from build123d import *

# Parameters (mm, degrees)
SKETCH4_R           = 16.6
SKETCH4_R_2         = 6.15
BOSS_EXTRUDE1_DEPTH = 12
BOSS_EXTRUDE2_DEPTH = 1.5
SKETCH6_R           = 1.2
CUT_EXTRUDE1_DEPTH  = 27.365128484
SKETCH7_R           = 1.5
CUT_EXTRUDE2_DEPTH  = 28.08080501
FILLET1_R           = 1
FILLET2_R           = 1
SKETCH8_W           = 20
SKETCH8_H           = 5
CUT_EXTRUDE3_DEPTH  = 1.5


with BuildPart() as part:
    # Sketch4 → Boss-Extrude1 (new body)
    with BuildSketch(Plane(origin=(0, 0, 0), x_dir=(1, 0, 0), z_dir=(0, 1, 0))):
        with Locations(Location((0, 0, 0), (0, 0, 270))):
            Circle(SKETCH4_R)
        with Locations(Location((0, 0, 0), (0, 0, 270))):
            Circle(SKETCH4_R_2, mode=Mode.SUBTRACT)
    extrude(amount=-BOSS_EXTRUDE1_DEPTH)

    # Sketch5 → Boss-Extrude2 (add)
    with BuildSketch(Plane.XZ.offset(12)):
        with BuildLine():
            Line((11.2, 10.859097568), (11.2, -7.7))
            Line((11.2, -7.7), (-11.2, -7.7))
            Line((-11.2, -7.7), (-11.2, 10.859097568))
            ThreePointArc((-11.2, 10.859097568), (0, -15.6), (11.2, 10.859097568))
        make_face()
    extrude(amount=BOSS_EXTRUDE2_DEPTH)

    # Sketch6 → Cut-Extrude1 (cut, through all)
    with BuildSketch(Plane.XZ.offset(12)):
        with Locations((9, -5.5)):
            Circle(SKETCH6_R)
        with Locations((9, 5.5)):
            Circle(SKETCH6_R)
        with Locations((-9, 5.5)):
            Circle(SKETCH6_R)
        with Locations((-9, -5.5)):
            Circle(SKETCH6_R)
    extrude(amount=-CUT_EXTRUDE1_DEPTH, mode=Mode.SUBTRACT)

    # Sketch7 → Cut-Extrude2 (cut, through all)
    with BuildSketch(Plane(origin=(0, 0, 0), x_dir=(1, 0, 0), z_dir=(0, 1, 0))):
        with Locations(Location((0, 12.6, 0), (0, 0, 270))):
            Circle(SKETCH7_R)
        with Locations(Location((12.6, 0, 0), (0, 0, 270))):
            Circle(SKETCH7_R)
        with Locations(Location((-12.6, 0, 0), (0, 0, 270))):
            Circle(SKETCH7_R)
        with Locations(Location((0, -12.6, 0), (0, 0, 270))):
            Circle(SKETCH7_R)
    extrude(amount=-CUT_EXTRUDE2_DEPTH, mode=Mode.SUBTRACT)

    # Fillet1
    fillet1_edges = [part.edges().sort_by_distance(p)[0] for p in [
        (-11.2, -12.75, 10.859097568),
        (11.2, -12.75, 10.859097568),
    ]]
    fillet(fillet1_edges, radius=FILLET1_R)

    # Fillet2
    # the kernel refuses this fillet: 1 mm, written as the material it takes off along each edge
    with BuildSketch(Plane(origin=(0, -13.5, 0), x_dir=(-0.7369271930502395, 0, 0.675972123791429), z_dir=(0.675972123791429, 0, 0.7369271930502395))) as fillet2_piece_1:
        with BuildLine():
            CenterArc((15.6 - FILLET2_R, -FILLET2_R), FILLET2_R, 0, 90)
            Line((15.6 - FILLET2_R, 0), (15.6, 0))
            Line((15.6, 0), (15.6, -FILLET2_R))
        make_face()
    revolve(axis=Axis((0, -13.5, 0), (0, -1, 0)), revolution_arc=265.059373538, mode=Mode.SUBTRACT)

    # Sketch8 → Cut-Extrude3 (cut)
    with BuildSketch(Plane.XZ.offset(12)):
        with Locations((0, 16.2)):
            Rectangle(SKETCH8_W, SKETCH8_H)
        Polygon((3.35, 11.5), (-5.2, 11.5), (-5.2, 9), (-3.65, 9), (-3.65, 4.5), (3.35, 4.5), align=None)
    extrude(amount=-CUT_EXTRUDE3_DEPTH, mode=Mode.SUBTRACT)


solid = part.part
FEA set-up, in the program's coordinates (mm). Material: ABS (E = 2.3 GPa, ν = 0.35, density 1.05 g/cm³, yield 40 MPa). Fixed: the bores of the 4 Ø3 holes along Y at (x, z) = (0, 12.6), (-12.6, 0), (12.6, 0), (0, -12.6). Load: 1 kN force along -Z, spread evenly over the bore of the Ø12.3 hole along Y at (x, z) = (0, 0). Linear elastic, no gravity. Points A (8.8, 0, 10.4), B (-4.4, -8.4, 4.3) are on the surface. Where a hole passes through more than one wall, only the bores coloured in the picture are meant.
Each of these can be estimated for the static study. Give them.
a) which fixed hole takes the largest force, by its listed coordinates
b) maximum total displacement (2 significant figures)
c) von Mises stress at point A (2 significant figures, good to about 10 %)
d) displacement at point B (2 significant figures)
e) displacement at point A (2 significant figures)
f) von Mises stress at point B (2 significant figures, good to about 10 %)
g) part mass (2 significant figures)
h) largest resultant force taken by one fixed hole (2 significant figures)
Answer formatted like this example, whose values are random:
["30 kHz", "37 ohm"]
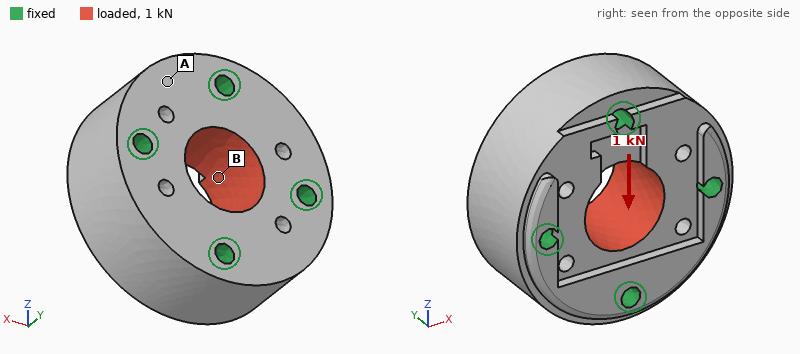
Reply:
["(0, -12.6)", "13 µm", "0.98 MPa", "12 µm", "7.6 µm", "3.2 MPa", "9.1 g", "310 N"]
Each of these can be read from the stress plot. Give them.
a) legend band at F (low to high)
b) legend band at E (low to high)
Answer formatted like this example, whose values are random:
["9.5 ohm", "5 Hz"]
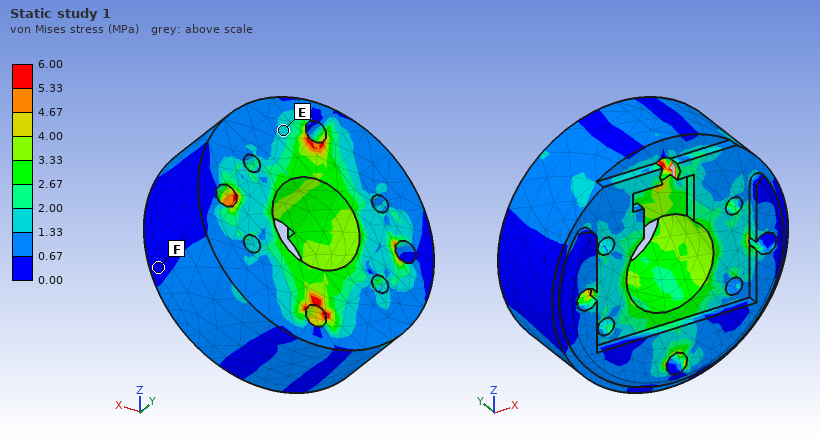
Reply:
["0.00 to 0.67 MPa", "1.33 to 2.00 MPa"]
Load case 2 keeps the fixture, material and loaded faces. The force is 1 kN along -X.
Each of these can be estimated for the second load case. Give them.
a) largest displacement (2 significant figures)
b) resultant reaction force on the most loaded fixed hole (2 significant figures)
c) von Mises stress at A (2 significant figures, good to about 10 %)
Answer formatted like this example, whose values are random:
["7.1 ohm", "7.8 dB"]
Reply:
["14 µm", "290 N", "1.00 MPa"]
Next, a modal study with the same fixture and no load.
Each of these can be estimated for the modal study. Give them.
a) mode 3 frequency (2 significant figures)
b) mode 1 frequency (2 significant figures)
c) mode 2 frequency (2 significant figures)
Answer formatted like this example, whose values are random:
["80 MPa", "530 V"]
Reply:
["19 kHz", "18 kHz", "19 kHz"]
